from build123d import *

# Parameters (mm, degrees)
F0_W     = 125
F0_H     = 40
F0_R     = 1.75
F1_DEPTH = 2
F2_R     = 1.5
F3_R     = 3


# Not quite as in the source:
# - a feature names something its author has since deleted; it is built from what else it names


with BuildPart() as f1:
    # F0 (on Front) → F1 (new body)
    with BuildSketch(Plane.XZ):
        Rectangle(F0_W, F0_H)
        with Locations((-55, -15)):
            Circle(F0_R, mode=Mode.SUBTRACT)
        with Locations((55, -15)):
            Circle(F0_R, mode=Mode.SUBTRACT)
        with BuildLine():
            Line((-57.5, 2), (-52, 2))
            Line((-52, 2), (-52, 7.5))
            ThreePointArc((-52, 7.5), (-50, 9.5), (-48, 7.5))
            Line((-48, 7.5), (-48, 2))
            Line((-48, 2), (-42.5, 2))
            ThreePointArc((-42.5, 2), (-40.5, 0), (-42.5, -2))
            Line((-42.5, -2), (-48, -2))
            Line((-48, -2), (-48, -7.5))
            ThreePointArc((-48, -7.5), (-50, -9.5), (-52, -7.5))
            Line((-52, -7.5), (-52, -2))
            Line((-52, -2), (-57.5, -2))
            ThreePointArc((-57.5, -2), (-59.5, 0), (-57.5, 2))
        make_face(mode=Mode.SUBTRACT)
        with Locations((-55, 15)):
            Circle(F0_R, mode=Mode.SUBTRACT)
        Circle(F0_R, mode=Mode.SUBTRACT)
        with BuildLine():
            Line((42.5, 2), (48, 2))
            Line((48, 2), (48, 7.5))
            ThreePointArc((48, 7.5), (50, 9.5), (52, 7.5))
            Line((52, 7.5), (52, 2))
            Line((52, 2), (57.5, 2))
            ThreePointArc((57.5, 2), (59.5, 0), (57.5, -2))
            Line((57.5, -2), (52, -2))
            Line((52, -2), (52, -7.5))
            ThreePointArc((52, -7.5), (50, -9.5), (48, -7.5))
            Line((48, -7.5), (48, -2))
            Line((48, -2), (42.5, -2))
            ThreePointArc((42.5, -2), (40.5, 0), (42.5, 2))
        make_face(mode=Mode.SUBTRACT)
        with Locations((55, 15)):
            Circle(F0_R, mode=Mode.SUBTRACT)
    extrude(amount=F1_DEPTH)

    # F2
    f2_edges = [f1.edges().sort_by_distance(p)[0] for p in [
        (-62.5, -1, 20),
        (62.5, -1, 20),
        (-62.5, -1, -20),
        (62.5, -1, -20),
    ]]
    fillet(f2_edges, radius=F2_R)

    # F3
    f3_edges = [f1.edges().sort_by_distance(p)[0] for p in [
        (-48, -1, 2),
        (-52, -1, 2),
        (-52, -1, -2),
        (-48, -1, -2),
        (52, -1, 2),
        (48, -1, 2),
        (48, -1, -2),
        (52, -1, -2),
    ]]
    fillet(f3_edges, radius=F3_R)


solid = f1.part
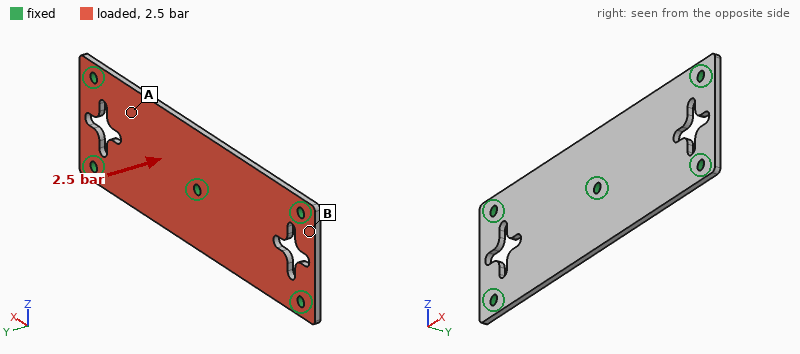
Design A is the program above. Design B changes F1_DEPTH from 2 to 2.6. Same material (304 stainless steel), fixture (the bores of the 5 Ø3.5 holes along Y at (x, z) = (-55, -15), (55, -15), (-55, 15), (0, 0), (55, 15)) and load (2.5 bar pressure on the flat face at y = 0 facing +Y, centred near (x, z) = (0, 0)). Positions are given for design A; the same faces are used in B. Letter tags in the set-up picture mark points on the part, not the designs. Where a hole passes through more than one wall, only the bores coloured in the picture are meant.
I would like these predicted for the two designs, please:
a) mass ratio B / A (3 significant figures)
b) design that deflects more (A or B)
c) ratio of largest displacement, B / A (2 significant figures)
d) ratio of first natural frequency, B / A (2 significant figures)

1.30
A
0.46
1.3
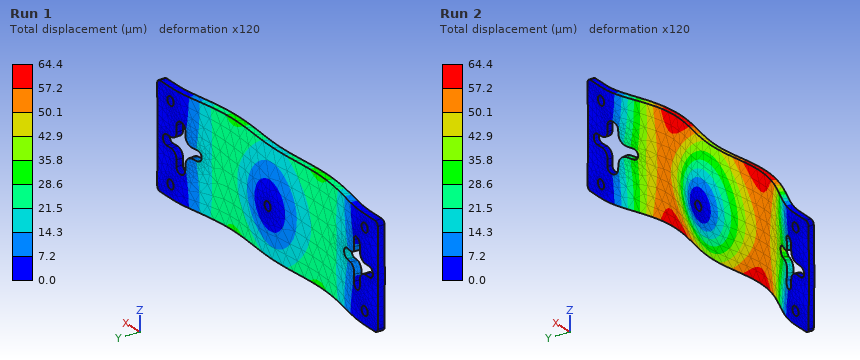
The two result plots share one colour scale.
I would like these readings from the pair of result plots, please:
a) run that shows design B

Run 1
